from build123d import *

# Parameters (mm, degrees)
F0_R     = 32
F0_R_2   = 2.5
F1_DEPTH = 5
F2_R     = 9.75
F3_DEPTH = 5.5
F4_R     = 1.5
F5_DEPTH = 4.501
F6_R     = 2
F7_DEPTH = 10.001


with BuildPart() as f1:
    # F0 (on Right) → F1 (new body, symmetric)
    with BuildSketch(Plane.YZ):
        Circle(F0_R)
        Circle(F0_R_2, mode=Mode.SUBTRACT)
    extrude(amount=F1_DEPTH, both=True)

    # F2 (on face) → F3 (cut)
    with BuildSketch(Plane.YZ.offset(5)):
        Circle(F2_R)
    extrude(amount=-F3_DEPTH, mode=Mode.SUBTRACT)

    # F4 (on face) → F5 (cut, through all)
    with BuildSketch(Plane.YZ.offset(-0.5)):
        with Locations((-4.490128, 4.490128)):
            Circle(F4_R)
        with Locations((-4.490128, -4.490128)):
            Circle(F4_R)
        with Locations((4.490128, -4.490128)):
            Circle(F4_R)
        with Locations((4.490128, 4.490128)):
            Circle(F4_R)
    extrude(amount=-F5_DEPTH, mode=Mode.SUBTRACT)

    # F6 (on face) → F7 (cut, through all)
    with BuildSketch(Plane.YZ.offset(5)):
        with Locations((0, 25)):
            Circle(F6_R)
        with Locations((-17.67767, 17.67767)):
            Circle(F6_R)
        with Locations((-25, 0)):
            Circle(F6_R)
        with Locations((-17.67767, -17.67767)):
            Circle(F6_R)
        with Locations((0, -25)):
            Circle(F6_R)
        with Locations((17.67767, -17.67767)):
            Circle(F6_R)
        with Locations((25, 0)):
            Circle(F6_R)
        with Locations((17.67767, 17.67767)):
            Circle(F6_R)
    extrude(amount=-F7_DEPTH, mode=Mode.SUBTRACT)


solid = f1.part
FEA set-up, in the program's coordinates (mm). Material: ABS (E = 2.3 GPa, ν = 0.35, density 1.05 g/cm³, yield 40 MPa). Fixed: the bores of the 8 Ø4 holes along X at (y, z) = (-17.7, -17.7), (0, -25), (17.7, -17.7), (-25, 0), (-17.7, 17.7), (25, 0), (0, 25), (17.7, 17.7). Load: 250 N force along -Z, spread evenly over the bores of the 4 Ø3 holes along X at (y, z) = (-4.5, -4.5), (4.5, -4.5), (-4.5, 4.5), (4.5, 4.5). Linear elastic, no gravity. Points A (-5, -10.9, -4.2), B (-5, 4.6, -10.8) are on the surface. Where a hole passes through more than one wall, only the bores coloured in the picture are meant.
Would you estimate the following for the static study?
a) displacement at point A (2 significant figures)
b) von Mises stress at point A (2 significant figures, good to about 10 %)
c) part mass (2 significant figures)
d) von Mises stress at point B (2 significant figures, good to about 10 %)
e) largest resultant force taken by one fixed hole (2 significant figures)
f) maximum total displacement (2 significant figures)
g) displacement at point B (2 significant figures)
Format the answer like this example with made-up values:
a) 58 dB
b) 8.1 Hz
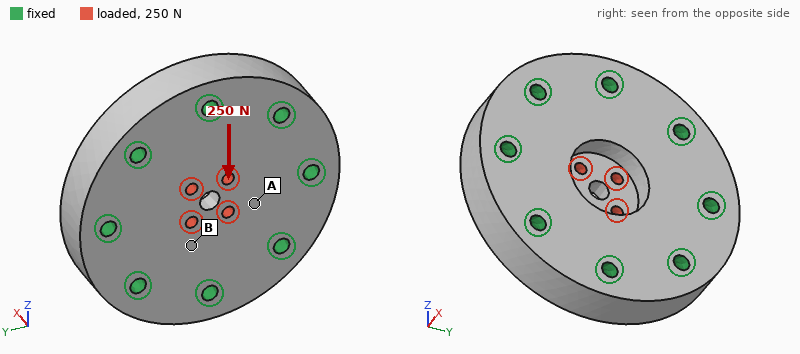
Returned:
a) 2.4 µm
b) 0.43 MPa
c) 31 g
d) 0.94 MPa
e) 53 N
f) 9.6 µm
g) 4.3 µm
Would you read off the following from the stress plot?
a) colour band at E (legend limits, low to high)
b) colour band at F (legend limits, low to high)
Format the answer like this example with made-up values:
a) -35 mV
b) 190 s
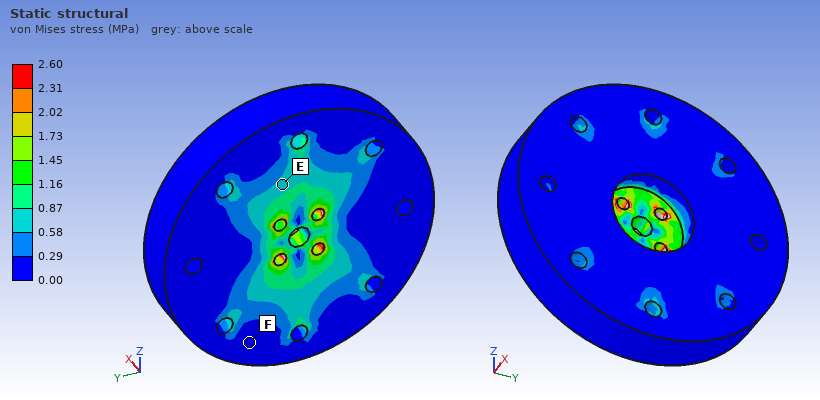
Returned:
a) 0.58 to 0.87 MPa
b) 0.00 to 0.29 MPa
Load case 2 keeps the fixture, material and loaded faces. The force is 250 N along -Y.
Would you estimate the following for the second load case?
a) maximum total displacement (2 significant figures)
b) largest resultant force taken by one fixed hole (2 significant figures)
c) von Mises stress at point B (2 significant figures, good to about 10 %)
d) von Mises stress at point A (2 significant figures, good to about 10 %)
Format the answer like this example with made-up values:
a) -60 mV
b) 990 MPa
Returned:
a) 9.5 µm
b) 53 N
c) 0.47 MPa
d) 0.94 MPa
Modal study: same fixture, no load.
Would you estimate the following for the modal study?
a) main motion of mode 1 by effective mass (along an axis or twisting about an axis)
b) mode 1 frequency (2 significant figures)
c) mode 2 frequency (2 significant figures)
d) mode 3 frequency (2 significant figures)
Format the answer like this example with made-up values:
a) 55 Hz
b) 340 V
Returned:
a) along X
b) 8600 Hz
c) 12 kHz
d) 12 kHz
